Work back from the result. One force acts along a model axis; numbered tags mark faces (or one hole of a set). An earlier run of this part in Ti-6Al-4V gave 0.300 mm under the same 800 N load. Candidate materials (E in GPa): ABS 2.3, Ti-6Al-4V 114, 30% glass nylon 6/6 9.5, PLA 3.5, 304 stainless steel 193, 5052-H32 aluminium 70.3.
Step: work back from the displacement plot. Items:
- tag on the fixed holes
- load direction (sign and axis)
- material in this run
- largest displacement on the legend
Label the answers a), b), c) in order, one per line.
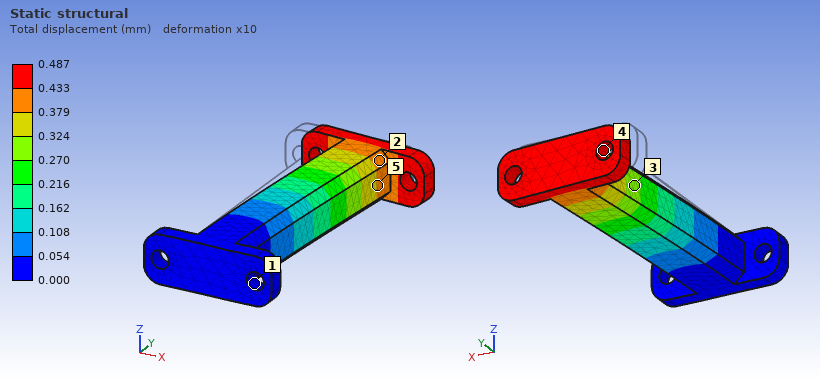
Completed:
a) 1
b) +X
c) 5052-H32 aluminium
d) 0.487 mm
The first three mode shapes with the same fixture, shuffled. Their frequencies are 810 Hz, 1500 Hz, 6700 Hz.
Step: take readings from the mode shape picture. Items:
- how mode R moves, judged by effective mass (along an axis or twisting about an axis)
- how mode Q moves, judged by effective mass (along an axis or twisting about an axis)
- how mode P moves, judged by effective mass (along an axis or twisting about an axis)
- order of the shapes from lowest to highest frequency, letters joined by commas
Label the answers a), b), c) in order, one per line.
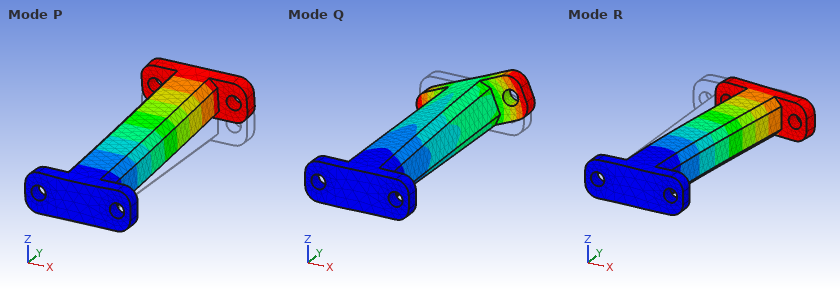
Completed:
a) along X
b) twisting about Y
c) along Z
d) P, R, Q
